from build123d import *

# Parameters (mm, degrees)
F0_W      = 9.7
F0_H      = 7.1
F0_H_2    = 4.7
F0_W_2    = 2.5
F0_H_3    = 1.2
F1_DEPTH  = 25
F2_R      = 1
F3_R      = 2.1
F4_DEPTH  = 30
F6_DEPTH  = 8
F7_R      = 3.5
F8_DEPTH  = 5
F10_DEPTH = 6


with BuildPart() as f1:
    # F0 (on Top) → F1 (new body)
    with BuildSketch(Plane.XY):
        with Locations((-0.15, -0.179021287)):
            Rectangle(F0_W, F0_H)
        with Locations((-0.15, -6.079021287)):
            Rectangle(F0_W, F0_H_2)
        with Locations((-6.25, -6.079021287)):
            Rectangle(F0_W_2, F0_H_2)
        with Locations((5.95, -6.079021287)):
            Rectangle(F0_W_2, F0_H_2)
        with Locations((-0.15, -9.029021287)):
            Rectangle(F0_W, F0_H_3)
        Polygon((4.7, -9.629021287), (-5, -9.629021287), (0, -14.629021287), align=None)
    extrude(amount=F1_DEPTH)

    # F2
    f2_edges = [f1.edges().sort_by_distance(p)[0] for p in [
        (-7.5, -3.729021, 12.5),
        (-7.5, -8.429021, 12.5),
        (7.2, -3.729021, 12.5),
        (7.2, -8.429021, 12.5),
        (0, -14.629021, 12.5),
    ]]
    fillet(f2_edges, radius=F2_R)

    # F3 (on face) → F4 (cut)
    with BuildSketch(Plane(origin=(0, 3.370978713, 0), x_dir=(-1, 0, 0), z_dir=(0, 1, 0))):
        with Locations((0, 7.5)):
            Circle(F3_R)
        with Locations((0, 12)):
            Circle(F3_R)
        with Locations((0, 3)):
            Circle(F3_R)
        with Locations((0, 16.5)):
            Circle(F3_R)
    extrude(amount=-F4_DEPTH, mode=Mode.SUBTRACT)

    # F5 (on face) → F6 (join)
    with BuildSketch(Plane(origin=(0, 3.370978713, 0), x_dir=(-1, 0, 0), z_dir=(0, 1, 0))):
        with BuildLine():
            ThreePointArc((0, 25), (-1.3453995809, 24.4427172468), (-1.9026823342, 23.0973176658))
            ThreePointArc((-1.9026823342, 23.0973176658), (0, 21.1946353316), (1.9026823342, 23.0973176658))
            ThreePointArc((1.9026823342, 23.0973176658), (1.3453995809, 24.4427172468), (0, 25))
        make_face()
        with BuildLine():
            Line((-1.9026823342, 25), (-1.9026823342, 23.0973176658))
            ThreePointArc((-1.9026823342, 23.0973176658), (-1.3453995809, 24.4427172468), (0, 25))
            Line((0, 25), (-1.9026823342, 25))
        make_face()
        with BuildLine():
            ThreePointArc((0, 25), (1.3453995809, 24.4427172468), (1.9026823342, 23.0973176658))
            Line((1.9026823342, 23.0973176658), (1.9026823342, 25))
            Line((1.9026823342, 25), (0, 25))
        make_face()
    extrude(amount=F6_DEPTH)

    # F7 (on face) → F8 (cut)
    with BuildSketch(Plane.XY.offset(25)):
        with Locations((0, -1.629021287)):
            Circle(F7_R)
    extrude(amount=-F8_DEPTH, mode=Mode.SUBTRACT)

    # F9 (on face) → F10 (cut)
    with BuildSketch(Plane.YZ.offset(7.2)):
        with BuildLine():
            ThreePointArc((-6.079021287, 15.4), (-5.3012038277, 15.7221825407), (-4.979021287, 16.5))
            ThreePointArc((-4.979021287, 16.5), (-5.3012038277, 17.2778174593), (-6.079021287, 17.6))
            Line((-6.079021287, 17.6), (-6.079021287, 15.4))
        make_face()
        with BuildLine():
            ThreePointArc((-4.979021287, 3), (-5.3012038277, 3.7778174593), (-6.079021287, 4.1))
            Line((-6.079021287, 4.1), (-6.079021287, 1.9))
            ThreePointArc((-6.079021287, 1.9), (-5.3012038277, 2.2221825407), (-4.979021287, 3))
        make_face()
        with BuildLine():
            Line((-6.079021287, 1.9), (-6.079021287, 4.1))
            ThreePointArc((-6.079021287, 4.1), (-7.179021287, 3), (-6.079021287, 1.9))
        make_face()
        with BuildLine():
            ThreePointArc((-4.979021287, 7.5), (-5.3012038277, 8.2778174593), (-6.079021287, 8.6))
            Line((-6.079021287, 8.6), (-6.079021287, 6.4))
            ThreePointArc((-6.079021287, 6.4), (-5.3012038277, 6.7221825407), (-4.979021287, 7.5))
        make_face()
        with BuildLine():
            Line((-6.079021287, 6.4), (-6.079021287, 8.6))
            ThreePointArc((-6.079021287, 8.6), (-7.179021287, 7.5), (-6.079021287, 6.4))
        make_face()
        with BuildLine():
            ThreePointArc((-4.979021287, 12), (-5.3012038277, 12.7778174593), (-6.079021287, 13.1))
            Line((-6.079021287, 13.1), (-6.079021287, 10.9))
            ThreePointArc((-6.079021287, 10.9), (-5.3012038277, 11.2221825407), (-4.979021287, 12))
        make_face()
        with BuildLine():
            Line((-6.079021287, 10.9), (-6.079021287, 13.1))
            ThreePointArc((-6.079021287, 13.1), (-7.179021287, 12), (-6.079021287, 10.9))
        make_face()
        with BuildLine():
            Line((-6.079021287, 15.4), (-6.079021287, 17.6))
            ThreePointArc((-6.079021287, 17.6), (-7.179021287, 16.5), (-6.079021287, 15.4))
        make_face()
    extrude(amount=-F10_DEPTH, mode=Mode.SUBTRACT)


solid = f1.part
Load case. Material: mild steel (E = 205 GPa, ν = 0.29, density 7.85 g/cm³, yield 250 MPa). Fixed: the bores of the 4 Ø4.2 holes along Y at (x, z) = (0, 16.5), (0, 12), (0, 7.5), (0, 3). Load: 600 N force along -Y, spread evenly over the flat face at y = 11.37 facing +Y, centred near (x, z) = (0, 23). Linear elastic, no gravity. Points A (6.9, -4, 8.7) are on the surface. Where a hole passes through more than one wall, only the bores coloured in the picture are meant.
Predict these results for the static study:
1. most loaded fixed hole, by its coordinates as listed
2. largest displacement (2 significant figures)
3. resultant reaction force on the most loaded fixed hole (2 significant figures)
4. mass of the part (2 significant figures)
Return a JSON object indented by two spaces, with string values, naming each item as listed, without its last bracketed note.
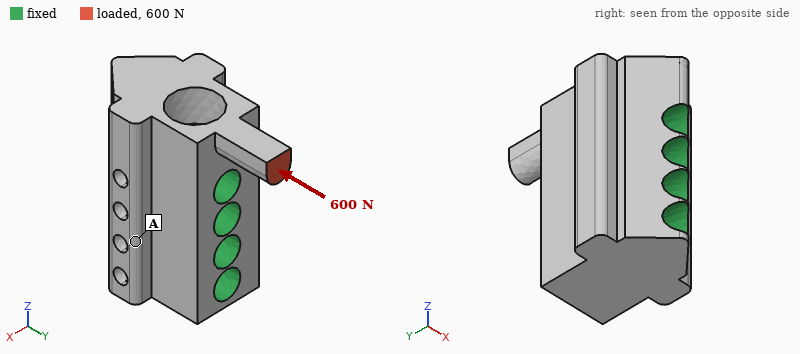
{
  "most loaded fixed hole, by its coordinates as listed": "(0, 16.5)",
  "largest displacement": "8.9 µm",
  "resultant reaction force on the most loaded fixed hole": "590 N",
  "mass of the part": "25 g"
}
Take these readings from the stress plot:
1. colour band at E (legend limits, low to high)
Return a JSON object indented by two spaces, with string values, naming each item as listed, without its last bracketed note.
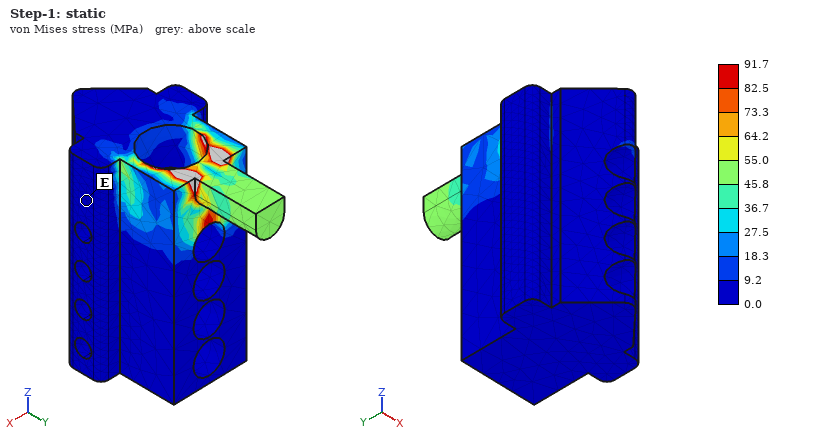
{
  "colour band at E": "0.0 to 9.2 MPa"
}
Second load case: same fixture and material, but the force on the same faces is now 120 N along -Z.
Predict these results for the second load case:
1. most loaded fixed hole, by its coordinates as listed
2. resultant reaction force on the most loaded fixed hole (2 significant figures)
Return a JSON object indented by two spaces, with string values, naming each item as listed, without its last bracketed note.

{
  "most loaded fixed hole, by its coordinates as listed": "(0, 16.5)",
  "resultant reaction force on the most loaded fixed hole": "140 N"
}
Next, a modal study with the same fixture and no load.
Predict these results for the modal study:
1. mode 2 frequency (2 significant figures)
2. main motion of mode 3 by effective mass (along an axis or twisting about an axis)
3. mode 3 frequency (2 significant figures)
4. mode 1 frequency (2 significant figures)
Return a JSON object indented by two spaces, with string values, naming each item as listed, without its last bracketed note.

{
  "mode 2 frequency": "28 kHz",
  "main motion of mode 3 by effective mass": "along X",
  "mode 3 frequency": "63 kHz",
  "mode 1 frequency": "25 kHz"
}
